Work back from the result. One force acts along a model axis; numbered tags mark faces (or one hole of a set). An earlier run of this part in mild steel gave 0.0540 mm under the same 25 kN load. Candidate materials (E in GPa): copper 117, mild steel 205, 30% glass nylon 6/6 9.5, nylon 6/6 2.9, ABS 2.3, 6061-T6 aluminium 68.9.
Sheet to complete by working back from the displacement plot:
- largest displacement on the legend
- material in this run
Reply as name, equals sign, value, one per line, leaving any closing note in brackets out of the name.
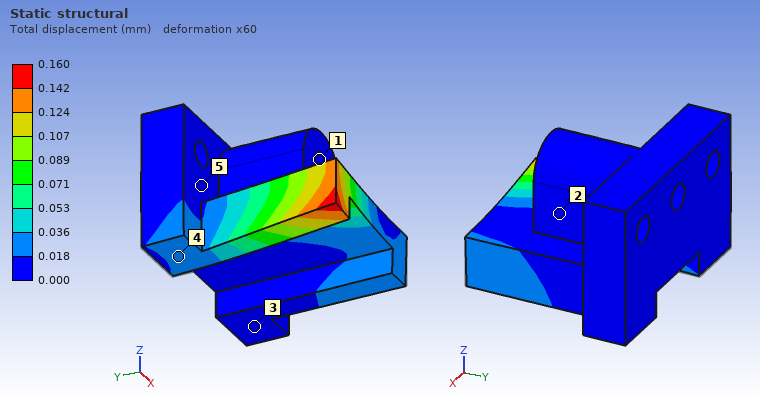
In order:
largest displacement on the legend = 0.160 mm
material in this run = 6061-T6 aluminium
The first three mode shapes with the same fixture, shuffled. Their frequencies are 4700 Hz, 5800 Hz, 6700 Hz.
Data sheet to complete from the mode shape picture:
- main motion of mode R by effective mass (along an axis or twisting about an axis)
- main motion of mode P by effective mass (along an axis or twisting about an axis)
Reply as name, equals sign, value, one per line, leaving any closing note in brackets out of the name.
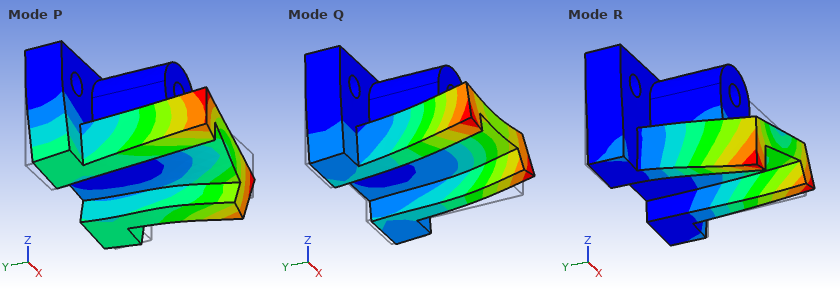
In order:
main motion of mode R by effective mass = along X
main motion of mode P by effective mass = twisting about Z
